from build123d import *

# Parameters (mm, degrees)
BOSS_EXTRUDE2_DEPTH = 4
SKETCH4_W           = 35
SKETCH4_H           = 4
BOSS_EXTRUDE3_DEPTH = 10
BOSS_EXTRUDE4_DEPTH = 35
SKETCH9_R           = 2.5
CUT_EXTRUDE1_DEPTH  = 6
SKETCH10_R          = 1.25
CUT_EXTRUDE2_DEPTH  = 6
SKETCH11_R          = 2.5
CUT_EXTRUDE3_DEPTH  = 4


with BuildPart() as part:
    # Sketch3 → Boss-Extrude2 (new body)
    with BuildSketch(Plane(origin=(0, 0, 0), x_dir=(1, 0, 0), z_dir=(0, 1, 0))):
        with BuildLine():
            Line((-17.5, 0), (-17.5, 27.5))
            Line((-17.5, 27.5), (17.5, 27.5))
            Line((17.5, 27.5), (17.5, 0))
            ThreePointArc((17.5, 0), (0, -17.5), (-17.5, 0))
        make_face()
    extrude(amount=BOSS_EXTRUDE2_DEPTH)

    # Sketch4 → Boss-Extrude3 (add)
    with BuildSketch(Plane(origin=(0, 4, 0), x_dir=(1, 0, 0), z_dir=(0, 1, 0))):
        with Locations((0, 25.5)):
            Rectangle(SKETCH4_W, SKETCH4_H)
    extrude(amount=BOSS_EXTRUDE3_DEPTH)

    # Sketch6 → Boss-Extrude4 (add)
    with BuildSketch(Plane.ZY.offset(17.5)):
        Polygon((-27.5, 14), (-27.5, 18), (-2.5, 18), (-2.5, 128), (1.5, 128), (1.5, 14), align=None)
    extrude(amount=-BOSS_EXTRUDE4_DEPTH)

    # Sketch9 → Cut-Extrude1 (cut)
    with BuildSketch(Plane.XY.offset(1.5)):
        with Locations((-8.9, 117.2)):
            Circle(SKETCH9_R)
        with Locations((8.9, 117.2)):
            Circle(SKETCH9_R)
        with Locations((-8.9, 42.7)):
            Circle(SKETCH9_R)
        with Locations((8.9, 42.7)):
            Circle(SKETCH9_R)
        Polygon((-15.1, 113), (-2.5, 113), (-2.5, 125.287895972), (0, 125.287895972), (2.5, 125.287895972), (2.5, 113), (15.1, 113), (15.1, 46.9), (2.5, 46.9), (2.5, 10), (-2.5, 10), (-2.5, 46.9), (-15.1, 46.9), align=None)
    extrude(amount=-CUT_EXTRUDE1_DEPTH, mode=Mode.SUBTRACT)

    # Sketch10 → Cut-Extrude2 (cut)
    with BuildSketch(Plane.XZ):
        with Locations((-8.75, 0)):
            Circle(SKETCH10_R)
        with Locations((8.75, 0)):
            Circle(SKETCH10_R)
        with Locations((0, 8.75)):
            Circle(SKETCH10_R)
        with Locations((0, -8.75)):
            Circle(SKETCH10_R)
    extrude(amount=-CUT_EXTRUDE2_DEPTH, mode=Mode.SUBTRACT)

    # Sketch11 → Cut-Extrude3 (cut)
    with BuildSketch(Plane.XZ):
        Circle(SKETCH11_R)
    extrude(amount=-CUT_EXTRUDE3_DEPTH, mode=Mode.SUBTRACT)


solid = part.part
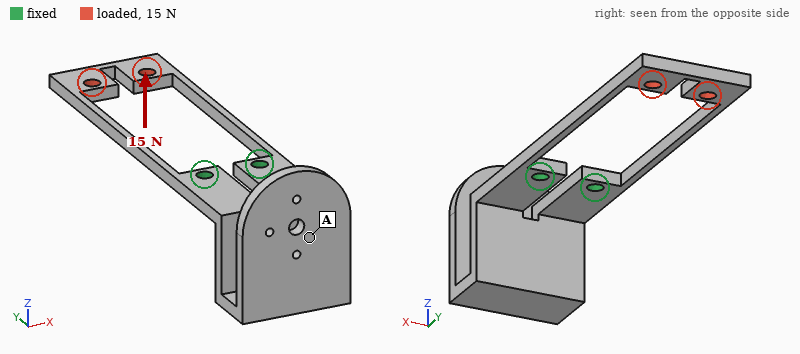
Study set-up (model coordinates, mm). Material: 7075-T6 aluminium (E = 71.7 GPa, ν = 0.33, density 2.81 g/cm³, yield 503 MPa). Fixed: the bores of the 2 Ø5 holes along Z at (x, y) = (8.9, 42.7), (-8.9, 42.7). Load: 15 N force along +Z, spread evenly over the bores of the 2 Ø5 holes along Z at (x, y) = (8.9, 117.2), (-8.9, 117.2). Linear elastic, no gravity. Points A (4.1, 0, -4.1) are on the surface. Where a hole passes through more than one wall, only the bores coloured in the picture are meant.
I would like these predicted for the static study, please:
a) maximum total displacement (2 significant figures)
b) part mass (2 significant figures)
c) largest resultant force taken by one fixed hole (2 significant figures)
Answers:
1.3 mm
48 g
7.5 N
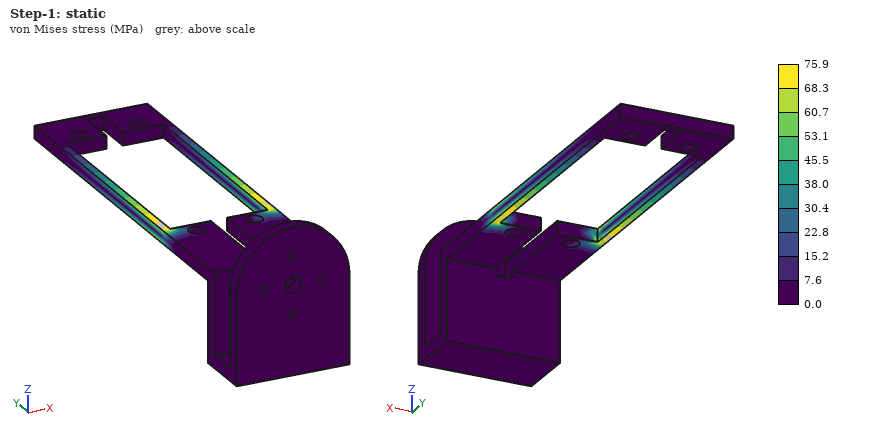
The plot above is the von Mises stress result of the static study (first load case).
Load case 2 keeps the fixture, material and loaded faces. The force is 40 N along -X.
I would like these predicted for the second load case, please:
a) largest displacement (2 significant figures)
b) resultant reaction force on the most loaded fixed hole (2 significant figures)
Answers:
1.7 mm
57 N
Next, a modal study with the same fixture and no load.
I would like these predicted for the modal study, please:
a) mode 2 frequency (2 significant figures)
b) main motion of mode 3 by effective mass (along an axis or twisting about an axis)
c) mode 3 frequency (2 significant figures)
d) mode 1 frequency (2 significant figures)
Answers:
320 Hz
along Z
630 Hz
240 Hz
